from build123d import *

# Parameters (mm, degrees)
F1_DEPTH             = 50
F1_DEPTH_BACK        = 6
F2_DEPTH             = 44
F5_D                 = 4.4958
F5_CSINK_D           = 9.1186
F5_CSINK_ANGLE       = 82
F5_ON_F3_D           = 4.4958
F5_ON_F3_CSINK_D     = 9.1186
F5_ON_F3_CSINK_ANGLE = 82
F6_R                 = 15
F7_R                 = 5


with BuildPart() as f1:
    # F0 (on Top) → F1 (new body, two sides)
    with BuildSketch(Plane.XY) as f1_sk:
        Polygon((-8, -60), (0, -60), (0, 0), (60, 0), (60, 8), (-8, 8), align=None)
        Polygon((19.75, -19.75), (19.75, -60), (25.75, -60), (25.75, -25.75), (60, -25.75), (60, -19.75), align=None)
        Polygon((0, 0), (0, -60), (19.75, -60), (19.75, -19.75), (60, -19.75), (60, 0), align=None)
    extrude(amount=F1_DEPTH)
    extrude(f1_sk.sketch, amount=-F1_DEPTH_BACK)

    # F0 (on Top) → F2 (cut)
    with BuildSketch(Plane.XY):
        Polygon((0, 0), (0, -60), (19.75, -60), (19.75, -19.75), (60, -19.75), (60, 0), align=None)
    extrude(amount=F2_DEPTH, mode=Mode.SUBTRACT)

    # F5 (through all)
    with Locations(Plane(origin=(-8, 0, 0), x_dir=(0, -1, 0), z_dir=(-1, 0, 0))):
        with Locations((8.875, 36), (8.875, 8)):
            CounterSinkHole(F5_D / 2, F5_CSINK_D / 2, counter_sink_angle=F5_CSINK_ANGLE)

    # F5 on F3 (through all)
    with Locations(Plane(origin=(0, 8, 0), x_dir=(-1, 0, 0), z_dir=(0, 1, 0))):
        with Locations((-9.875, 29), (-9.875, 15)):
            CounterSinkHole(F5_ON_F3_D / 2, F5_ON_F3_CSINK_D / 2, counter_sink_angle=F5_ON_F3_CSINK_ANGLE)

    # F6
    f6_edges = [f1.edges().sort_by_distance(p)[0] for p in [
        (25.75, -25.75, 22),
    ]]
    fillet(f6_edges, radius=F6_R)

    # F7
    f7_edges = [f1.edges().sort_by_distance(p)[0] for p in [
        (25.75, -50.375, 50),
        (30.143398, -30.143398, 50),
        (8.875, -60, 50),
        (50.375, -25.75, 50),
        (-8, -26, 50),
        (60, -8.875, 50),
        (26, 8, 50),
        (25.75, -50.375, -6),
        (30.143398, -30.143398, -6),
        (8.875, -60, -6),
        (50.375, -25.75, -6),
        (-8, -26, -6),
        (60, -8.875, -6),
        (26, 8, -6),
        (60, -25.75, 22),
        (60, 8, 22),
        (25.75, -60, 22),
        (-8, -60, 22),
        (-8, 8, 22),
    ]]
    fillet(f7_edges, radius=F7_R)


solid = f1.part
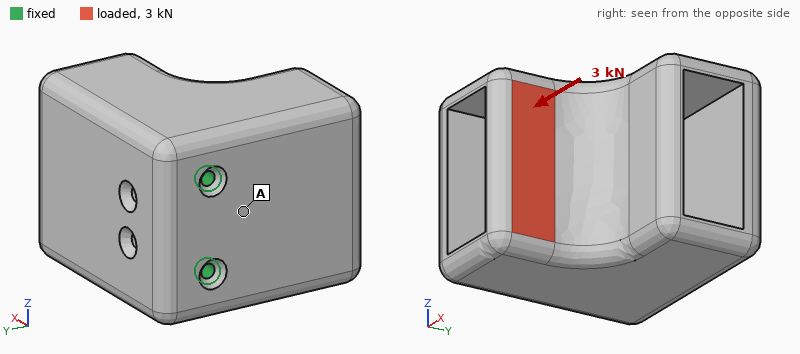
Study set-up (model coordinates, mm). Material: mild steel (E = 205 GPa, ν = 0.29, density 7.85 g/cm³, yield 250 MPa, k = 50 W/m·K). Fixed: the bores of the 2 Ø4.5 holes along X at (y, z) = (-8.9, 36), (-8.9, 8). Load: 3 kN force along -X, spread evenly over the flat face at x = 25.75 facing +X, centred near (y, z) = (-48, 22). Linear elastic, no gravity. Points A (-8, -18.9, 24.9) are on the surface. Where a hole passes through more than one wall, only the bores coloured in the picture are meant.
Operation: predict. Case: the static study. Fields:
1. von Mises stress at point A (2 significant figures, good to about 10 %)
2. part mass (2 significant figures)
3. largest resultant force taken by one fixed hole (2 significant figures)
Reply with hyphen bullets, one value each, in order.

- 44 MPa
- 820 g
- 1.5 kN
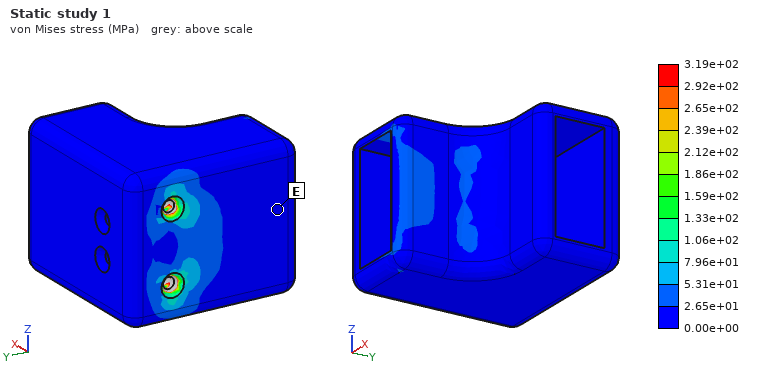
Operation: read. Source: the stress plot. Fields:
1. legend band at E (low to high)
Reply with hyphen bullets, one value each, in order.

- 0.00e+00 to 2.65e+01 MPa
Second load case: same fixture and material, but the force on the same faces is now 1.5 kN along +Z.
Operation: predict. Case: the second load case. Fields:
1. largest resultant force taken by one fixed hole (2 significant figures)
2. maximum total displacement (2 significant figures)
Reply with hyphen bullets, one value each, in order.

- 2.4 kN
- 18 µm
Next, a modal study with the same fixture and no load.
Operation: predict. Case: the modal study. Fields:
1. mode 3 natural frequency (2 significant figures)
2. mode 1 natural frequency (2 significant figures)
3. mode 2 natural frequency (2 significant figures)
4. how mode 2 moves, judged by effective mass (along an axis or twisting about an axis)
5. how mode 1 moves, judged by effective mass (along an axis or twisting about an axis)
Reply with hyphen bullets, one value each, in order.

- 4600 Hz
- 1000 Hz
- 2500 Hz
- along Z
- along Y
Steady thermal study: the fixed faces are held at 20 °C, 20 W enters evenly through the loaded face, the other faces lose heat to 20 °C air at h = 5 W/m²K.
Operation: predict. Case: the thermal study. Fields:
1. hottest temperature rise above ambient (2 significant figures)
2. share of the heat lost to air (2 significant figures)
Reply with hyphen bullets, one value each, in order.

- 40 K
- 12 %
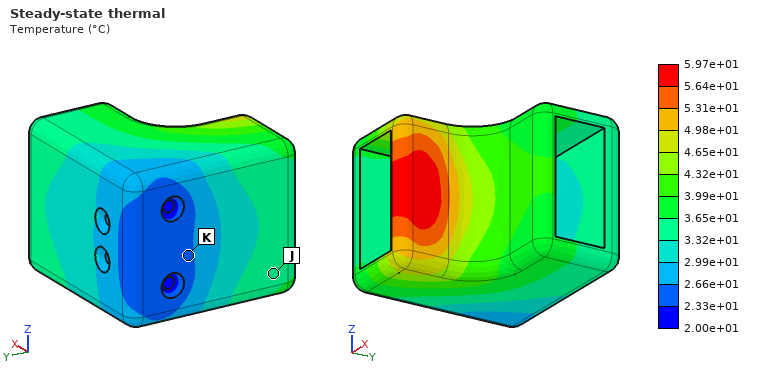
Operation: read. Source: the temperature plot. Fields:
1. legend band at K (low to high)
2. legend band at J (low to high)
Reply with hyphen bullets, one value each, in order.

- 2.33e+01 to 2.66e+01 °C
- 3.32e+01 to 3.65e+01 °C
